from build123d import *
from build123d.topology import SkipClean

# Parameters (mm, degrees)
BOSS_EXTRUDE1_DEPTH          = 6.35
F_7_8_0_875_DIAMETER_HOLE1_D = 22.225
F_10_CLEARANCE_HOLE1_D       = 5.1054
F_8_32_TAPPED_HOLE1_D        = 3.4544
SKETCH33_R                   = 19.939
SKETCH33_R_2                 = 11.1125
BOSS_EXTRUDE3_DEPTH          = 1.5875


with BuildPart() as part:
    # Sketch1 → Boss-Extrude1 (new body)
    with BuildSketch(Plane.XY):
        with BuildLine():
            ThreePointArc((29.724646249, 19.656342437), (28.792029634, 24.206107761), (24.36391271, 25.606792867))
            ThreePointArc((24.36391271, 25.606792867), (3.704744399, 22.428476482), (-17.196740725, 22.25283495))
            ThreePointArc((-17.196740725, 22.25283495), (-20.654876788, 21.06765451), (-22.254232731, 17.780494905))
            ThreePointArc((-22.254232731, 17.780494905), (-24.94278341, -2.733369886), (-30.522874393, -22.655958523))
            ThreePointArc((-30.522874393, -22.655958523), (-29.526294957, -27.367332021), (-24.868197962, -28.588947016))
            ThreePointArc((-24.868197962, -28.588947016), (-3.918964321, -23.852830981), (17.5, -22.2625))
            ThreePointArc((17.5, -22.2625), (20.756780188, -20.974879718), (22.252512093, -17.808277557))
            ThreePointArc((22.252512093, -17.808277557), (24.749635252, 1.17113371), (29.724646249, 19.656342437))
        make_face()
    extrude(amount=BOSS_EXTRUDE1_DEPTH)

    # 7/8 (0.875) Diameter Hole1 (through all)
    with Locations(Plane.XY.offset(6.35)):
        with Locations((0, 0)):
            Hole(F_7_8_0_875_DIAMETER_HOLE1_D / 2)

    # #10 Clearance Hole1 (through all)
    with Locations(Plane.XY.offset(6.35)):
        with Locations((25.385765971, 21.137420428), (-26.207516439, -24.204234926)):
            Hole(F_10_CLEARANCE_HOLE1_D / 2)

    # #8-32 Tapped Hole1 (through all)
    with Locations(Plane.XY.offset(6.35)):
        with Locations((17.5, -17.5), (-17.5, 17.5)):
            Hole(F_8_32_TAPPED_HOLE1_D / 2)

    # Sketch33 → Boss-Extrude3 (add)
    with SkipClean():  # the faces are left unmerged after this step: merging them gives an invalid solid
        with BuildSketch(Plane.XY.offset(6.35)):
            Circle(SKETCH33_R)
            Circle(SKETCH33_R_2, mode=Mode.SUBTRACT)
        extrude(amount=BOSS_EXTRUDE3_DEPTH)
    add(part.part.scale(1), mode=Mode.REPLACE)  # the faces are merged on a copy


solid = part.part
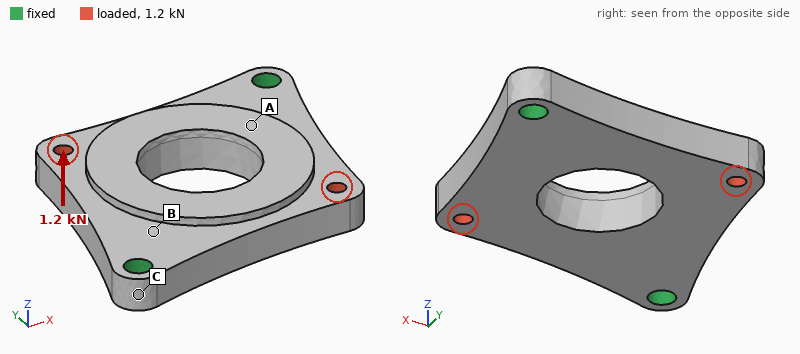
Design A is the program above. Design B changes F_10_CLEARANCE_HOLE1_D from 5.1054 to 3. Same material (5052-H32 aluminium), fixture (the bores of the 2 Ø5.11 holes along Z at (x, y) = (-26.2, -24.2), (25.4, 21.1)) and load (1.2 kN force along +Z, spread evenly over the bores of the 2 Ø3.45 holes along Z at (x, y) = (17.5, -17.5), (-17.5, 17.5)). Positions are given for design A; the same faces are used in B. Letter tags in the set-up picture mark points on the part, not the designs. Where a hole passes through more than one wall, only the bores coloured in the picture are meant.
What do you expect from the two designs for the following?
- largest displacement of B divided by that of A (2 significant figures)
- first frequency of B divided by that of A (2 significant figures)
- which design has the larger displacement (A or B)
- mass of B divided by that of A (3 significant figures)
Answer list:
1.1
0.91
B
1.01
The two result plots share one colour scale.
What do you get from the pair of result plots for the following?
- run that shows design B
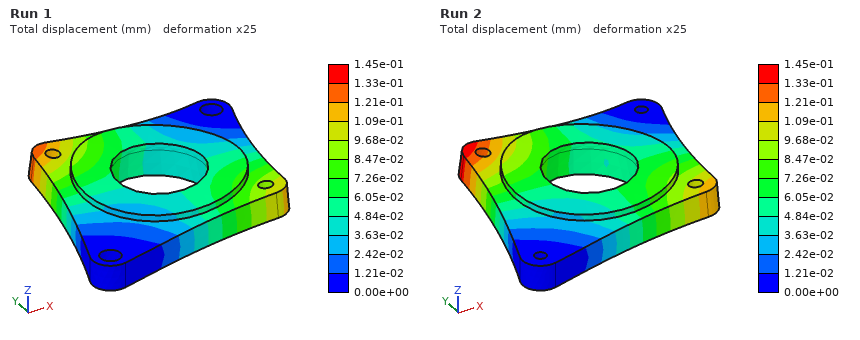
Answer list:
Run 2
